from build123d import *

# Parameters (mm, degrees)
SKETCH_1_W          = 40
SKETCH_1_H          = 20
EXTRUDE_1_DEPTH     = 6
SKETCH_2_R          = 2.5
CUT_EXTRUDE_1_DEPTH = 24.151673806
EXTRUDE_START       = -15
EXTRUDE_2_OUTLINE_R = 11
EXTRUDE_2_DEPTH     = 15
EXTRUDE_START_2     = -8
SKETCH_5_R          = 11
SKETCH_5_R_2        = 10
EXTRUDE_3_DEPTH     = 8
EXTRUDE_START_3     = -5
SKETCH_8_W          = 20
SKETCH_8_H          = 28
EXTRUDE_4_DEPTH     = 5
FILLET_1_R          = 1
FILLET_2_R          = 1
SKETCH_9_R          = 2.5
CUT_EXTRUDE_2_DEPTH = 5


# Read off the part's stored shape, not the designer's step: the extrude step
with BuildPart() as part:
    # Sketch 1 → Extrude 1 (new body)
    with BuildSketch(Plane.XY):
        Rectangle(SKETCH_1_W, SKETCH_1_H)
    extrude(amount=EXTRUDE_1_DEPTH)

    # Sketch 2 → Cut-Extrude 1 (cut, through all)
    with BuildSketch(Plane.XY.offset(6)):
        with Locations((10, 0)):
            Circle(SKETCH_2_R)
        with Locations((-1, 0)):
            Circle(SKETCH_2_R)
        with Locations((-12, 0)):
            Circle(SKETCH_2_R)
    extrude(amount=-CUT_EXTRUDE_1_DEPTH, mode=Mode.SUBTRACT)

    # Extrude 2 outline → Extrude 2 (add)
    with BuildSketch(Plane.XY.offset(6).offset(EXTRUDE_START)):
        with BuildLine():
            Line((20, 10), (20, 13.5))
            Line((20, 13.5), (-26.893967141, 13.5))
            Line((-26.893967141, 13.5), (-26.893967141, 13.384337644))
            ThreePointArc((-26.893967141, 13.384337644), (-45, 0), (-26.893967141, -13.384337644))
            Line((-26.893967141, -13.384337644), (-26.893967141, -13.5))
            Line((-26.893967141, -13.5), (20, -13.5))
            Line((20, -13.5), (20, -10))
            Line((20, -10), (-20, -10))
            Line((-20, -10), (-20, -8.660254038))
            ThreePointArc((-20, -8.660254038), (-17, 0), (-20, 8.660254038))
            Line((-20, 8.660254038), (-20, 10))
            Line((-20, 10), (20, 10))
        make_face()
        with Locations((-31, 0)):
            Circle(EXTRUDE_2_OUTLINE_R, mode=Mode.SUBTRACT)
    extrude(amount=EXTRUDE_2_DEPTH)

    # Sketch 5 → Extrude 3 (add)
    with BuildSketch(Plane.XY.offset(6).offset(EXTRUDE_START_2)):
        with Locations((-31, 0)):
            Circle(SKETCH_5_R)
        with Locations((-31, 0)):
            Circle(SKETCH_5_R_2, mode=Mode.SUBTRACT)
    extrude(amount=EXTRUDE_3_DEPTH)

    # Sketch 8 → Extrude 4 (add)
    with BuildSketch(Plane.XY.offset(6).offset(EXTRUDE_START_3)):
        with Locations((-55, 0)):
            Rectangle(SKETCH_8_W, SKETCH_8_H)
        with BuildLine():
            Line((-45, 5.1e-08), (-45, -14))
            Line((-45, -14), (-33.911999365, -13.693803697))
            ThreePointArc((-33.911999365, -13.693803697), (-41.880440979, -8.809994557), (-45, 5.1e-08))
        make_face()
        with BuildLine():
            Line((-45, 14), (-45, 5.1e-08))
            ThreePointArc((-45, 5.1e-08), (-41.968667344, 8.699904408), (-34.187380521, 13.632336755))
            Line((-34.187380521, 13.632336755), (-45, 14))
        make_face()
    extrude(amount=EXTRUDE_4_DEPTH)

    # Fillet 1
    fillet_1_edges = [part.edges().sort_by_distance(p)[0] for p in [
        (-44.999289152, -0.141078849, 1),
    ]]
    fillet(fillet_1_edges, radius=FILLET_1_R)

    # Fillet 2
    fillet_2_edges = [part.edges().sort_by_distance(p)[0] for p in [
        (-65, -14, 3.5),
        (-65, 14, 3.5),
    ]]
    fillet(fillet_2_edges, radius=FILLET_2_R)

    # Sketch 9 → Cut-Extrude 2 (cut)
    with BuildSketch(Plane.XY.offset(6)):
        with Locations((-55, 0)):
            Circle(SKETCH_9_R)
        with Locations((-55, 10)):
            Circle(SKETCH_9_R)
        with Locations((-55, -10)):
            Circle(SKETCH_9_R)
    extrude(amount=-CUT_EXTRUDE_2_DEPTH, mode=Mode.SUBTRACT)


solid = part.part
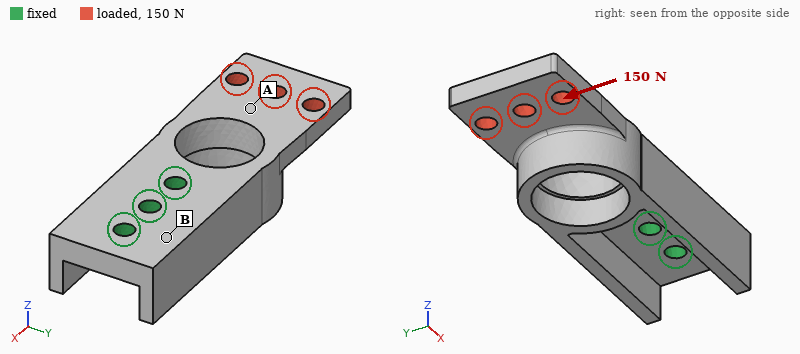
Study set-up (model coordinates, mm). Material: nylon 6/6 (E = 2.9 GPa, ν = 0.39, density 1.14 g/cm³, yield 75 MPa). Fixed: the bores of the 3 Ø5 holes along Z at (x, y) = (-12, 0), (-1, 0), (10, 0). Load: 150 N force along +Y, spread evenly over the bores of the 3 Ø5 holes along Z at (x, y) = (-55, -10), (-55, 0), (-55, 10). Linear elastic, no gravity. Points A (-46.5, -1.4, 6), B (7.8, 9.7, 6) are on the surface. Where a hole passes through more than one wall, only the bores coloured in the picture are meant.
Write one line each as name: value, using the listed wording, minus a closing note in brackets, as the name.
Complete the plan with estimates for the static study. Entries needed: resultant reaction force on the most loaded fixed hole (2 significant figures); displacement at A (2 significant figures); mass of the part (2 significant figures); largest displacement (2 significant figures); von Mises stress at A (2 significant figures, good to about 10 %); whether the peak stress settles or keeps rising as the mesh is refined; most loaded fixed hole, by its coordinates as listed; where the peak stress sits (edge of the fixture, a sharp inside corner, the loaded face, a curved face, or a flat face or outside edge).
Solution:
resultant reaction force on the most loaded fixed hole: 400 N
displacement at A: 0.33 mm
mass of the part: 18 g
largest displacement: 0.47 mm
von Mises stress at A: 3.5 MPa
whether the peak stress settles or keeps rising as the mesh is refined: keeps rising
most loaded fixed hole, by its coordinates as listed: (-12, 0)
where the peak stress sits: edge of the fixture
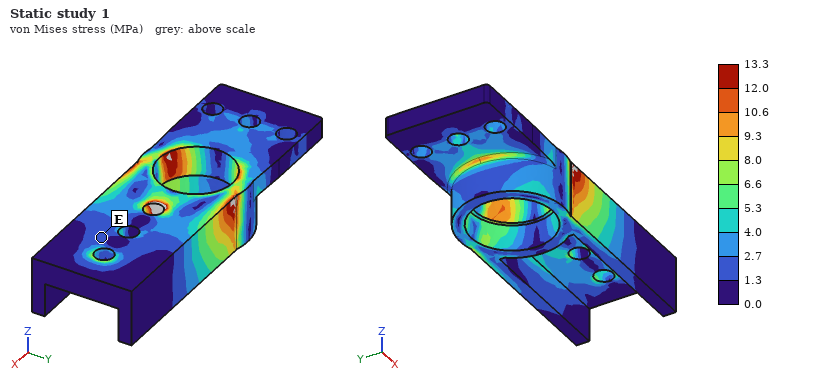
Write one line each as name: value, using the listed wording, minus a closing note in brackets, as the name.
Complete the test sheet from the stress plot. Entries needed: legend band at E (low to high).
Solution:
legend band at E: 1.3 to 2.7 MPa
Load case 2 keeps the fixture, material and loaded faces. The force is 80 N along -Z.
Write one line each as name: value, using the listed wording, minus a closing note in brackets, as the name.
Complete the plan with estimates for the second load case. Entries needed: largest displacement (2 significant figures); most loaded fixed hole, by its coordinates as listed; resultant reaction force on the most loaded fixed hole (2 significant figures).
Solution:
largest displacement: 0.91 mm
most loaded fixed hole, by its coordinates as listed: (-12, 0)
resultant reaction force on the most loaded fixed hole: 200 N
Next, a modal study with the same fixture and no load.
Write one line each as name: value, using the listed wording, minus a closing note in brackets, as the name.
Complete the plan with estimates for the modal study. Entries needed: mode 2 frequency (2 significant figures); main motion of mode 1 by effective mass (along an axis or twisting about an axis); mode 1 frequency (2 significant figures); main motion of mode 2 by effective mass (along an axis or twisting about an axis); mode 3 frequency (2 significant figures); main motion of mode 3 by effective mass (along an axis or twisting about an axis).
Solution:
mode 2 frequency: 1500 Hz
main motion of mode 1 by effective mass: along Z
mode 1 frequency: 930 Hz
main motion of mode 2 by effective mass: along Y
mode 3 frequency: 1900 Hz
main motion of mode 3 by effective mass: twisting about X
